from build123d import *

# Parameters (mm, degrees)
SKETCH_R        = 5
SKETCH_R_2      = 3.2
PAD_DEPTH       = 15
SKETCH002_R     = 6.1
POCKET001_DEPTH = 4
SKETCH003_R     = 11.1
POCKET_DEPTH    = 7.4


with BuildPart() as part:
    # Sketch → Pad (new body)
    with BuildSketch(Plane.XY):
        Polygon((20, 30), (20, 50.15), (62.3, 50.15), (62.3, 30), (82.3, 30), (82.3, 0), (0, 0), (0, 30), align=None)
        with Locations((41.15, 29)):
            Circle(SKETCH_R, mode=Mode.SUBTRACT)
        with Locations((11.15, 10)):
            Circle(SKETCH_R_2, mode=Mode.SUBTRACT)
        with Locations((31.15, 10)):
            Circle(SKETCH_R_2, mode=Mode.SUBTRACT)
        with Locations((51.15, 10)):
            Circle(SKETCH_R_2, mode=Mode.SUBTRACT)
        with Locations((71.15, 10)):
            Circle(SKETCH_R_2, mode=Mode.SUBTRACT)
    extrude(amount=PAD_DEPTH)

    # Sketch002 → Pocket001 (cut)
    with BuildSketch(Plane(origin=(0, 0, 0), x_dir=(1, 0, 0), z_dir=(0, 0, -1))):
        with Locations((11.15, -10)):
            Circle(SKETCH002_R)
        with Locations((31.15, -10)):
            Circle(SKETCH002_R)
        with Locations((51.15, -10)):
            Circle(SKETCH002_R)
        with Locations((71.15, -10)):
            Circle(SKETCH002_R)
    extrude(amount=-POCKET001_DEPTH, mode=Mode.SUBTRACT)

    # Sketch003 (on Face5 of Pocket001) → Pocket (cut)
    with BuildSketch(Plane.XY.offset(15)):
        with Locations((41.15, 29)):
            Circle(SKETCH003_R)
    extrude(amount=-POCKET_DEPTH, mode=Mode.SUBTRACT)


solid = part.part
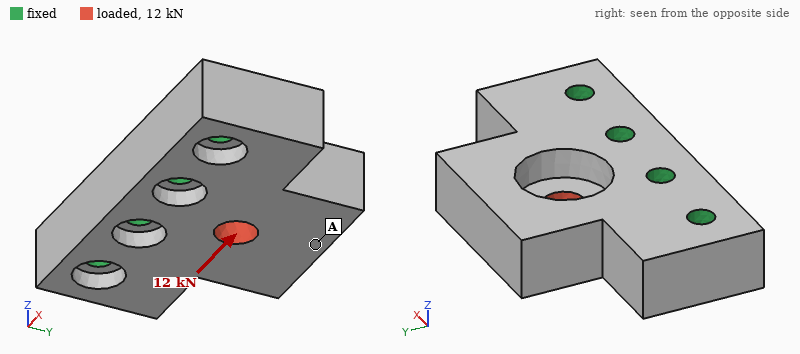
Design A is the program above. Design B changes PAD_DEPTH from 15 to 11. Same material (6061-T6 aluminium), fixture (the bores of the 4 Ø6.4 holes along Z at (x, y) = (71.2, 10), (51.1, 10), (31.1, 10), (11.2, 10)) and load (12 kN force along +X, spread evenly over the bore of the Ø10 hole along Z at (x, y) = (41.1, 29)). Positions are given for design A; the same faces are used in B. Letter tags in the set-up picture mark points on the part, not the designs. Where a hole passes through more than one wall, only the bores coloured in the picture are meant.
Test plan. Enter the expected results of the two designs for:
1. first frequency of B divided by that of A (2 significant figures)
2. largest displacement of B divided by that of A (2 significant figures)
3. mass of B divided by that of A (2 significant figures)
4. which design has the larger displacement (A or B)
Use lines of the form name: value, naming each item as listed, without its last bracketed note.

first frequency of B divided by that of A: 0.76
largest displacement of B divided by that of A: 1.2
mass of B divided by that of A: 0.74
which design has the larger displacement: B
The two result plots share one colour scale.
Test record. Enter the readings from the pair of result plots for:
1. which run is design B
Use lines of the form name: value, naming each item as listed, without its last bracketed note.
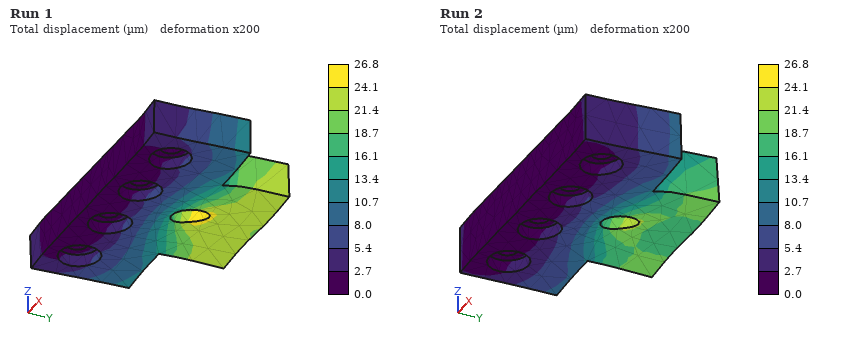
which run is design B: Run 1
